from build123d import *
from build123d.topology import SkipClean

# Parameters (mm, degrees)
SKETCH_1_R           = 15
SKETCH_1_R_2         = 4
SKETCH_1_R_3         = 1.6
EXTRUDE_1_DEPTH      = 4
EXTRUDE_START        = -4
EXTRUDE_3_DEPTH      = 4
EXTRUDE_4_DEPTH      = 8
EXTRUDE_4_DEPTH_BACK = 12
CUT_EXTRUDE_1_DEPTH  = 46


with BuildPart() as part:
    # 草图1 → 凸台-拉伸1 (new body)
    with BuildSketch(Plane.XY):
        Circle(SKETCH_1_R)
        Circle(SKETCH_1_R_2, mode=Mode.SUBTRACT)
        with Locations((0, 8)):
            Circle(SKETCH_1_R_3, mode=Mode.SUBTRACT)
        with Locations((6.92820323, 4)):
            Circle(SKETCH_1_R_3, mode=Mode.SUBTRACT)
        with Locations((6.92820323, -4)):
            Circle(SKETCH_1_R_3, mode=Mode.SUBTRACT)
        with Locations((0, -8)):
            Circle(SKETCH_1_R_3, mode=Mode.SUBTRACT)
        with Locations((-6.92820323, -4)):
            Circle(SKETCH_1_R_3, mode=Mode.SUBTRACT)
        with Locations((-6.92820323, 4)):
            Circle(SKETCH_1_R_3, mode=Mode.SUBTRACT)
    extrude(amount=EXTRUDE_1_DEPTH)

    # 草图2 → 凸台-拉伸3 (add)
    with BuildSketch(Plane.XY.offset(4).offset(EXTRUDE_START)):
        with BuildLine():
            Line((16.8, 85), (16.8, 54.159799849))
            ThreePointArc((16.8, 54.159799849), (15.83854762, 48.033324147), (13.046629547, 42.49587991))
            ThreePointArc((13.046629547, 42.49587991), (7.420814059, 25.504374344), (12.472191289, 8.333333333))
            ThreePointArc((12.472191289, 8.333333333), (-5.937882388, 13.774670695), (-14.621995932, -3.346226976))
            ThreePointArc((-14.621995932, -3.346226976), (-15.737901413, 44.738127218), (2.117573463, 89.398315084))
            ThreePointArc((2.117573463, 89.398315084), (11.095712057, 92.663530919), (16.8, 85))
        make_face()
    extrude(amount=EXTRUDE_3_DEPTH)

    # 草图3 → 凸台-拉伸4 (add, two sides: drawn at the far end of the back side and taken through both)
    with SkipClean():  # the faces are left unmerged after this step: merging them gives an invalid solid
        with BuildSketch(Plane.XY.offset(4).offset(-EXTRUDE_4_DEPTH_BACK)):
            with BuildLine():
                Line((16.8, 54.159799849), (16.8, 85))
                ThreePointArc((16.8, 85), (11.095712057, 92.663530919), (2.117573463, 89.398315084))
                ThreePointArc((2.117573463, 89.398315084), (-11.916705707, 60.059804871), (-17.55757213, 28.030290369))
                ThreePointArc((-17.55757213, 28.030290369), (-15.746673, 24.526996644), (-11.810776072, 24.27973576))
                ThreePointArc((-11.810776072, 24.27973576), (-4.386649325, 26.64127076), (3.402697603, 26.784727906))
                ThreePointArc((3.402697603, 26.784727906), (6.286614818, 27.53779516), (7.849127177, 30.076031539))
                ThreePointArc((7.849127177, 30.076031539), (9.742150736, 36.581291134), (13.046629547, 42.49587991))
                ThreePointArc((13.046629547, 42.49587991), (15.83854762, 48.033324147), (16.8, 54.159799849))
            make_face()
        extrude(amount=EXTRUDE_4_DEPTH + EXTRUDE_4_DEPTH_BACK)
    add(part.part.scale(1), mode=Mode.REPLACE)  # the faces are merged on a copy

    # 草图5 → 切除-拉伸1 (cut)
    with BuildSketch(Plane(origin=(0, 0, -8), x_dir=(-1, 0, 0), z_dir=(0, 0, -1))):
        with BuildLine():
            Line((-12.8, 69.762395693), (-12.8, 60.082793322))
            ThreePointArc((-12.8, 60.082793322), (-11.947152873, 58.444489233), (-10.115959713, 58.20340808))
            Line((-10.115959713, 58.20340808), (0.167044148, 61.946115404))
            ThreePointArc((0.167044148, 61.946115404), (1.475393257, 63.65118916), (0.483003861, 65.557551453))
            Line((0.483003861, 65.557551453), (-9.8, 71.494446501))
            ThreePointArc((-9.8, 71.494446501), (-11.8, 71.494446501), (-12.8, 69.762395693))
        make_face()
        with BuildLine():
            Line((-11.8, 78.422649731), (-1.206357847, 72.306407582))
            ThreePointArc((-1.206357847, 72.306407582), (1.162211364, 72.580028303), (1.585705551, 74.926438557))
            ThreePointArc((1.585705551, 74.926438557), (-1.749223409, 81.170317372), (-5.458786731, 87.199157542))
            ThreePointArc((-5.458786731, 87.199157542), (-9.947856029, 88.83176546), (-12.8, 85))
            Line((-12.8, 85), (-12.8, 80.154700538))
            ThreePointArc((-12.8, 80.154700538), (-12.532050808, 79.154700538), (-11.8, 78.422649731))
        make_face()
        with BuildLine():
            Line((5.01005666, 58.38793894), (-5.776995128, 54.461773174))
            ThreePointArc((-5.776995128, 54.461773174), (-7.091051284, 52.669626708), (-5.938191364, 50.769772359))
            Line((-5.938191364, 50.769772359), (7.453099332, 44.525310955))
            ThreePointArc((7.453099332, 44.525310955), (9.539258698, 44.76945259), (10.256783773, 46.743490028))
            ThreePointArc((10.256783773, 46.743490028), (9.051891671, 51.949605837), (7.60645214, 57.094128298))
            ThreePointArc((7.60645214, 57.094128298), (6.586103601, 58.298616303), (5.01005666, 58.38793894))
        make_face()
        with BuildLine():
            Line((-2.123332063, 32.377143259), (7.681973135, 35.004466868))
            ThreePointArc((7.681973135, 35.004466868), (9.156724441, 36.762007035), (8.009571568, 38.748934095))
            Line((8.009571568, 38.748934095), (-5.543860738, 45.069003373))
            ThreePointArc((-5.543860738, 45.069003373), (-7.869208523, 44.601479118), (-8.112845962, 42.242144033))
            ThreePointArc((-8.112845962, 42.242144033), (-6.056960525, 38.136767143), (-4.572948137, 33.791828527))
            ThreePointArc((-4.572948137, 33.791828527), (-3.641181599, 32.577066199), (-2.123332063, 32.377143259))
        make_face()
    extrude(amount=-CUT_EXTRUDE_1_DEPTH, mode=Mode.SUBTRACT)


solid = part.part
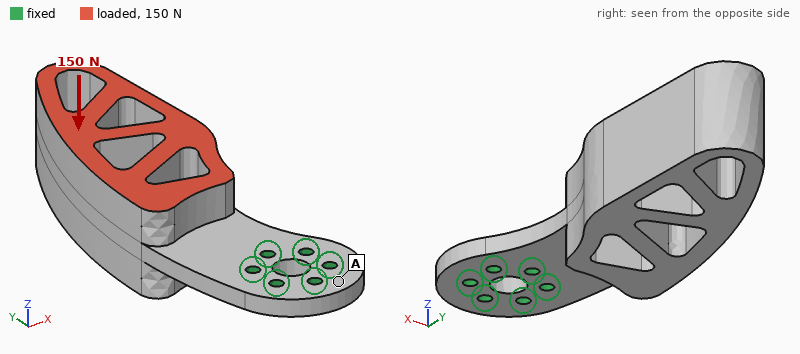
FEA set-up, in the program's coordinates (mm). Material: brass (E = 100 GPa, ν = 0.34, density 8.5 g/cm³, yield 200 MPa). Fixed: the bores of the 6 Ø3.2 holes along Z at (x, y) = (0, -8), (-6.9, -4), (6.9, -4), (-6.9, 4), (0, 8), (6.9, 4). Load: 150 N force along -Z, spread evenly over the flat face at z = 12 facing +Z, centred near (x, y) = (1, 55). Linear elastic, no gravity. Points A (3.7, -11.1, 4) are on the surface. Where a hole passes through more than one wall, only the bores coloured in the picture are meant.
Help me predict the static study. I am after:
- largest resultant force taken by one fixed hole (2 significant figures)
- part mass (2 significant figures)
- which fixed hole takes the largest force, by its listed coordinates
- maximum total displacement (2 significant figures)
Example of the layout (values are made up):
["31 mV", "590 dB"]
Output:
["490 N", "220 g", "(0, 8)", "0.59 mm"]
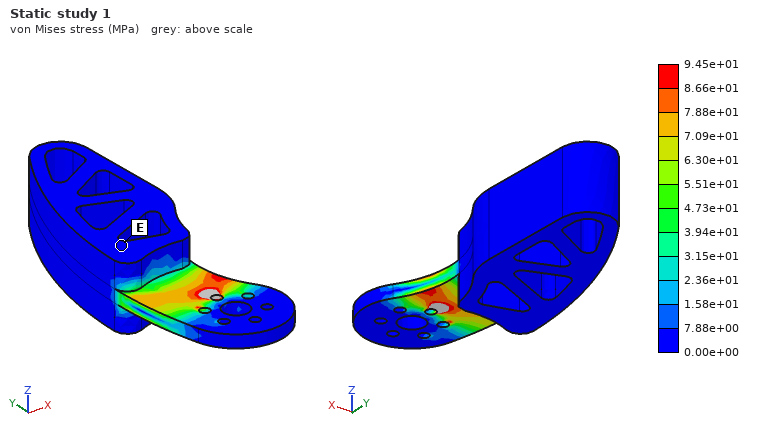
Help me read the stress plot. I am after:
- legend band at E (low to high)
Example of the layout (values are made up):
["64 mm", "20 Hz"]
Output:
["0.00e+00 to 7.88e+00 MPa"]
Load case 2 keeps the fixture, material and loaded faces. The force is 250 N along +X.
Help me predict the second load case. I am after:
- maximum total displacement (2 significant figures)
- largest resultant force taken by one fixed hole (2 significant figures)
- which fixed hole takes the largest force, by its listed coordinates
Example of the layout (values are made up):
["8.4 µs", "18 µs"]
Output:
["61 µm", "510 N", "(-6.9, 4)"]
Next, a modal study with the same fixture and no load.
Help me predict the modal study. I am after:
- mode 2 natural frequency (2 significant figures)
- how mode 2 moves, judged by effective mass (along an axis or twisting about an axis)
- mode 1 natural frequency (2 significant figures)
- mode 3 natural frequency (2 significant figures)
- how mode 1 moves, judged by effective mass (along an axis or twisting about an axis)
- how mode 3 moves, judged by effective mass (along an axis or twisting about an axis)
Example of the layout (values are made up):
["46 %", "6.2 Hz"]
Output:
["1100 Hz", "along X", "230 Hz", "1300 Hz", "along Z", "twisting about Y"]
